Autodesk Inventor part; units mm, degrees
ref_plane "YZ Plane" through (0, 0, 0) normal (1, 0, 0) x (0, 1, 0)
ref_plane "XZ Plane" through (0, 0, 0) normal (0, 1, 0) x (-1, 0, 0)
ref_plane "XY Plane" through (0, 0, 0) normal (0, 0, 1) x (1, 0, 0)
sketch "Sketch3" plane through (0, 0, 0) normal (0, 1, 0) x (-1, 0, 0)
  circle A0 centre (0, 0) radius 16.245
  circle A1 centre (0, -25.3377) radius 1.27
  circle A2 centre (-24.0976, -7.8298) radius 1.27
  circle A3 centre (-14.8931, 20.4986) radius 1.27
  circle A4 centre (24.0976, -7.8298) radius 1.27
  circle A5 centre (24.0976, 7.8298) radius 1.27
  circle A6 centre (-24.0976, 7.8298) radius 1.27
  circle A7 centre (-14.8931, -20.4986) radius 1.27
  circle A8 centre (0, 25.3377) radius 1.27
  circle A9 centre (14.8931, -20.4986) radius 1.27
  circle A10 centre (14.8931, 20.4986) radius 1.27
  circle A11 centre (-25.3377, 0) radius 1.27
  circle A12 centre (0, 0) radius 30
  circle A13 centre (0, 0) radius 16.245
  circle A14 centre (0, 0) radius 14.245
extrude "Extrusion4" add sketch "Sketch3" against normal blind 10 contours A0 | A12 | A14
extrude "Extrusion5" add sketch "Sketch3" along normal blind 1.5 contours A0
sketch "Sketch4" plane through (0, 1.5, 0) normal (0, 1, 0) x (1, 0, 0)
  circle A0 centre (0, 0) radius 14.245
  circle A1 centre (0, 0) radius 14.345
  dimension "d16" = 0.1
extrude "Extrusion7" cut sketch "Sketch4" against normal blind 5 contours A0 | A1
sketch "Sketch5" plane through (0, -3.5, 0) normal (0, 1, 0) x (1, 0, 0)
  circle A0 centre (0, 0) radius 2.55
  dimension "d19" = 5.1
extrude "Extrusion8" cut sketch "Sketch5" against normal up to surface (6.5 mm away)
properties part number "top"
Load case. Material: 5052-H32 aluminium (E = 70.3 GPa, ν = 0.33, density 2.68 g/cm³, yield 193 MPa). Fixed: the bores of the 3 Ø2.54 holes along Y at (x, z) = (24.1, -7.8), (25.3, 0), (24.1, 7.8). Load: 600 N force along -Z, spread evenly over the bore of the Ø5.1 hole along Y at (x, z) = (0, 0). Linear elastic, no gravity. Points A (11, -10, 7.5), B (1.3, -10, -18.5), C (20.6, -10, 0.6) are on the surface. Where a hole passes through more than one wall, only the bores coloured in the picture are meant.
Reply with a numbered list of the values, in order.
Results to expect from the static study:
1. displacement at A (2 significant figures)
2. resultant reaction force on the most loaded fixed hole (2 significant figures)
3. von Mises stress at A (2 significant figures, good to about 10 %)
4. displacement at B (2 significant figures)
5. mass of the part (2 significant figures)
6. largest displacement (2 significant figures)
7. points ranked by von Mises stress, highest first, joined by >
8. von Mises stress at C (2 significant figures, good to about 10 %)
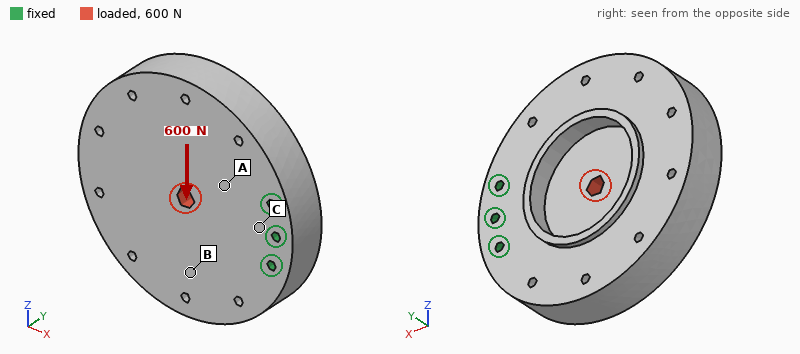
1. 3.3 µm
2. 850 N
3. 5.5 MPa
4. 6.5 µm
5. 69 g
6. 11 µm
7. C > A > B
8. 7.1 MPa
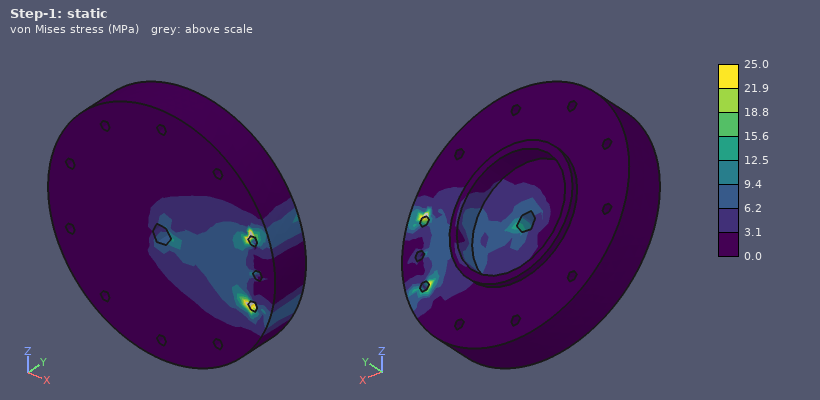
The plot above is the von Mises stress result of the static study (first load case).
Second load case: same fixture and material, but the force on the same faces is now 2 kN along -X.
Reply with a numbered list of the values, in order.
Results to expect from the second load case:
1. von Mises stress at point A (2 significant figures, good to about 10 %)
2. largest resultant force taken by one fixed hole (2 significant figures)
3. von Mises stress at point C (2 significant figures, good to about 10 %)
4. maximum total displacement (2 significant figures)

1. 10 MPa
2. 790 N
3. 13 MPa
4. 13 µm
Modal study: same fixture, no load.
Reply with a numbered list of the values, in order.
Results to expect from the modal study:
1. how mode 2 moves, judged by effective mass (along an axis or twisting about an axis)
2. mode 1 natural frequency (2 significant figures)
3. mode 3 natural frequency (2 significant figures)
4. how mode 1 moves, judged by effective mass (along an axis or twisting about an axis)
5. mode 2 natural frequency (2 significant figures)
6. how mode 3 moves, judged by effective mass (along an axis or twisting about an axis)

1. along Z
2. 2500 Hz
3. 5200 Hz
4. along Y
5. 4700 Hz
6. along Z
